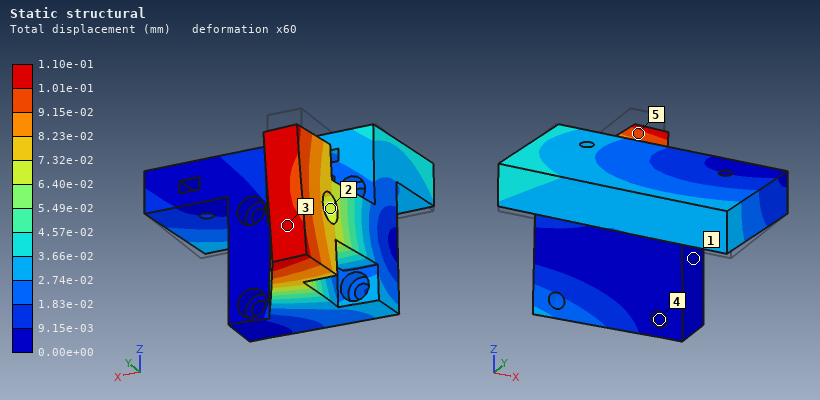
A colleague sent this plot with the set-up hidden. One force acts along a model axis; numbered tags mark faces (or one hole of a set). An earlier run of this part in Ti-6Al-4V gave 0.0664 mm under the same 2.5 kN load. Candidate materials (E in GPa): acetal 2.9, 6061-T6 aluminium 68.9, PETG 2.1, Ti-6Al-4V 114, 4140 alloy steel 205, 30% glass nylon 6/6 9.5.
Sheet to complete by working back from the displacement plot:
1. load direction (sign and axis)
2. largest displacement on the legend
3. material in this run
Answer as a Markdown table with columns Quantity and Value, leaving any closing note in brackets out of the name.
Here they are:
| Quantity | Value |
|---|---|
| load direction | -Z |
| largest displacement on the legend | 1.10e-01 mm |
| material in this run | 6061-T6 aluminium |
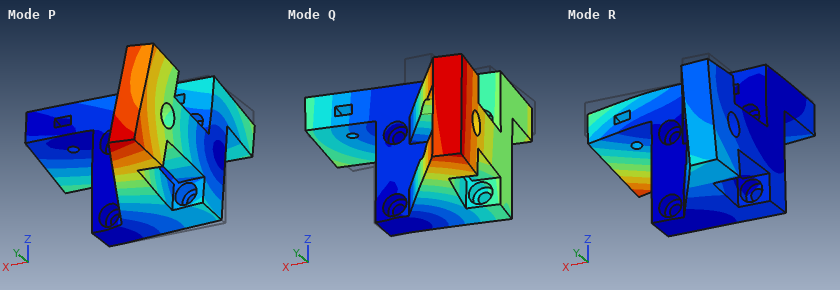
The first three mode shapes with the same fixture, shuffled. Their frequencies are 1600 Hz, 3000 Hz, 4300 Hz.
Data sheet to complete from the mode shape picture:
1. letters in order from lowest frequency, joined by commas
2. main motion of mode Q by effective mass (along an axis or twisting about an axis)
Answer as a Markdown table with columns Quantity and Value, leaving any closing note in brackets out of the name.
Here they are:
| Quantity | Value |
|---|---|
| letters in order from lowest frequency, joined by commas | Q, P, R |
| main motion of mode Q by effective mass | along Y |
